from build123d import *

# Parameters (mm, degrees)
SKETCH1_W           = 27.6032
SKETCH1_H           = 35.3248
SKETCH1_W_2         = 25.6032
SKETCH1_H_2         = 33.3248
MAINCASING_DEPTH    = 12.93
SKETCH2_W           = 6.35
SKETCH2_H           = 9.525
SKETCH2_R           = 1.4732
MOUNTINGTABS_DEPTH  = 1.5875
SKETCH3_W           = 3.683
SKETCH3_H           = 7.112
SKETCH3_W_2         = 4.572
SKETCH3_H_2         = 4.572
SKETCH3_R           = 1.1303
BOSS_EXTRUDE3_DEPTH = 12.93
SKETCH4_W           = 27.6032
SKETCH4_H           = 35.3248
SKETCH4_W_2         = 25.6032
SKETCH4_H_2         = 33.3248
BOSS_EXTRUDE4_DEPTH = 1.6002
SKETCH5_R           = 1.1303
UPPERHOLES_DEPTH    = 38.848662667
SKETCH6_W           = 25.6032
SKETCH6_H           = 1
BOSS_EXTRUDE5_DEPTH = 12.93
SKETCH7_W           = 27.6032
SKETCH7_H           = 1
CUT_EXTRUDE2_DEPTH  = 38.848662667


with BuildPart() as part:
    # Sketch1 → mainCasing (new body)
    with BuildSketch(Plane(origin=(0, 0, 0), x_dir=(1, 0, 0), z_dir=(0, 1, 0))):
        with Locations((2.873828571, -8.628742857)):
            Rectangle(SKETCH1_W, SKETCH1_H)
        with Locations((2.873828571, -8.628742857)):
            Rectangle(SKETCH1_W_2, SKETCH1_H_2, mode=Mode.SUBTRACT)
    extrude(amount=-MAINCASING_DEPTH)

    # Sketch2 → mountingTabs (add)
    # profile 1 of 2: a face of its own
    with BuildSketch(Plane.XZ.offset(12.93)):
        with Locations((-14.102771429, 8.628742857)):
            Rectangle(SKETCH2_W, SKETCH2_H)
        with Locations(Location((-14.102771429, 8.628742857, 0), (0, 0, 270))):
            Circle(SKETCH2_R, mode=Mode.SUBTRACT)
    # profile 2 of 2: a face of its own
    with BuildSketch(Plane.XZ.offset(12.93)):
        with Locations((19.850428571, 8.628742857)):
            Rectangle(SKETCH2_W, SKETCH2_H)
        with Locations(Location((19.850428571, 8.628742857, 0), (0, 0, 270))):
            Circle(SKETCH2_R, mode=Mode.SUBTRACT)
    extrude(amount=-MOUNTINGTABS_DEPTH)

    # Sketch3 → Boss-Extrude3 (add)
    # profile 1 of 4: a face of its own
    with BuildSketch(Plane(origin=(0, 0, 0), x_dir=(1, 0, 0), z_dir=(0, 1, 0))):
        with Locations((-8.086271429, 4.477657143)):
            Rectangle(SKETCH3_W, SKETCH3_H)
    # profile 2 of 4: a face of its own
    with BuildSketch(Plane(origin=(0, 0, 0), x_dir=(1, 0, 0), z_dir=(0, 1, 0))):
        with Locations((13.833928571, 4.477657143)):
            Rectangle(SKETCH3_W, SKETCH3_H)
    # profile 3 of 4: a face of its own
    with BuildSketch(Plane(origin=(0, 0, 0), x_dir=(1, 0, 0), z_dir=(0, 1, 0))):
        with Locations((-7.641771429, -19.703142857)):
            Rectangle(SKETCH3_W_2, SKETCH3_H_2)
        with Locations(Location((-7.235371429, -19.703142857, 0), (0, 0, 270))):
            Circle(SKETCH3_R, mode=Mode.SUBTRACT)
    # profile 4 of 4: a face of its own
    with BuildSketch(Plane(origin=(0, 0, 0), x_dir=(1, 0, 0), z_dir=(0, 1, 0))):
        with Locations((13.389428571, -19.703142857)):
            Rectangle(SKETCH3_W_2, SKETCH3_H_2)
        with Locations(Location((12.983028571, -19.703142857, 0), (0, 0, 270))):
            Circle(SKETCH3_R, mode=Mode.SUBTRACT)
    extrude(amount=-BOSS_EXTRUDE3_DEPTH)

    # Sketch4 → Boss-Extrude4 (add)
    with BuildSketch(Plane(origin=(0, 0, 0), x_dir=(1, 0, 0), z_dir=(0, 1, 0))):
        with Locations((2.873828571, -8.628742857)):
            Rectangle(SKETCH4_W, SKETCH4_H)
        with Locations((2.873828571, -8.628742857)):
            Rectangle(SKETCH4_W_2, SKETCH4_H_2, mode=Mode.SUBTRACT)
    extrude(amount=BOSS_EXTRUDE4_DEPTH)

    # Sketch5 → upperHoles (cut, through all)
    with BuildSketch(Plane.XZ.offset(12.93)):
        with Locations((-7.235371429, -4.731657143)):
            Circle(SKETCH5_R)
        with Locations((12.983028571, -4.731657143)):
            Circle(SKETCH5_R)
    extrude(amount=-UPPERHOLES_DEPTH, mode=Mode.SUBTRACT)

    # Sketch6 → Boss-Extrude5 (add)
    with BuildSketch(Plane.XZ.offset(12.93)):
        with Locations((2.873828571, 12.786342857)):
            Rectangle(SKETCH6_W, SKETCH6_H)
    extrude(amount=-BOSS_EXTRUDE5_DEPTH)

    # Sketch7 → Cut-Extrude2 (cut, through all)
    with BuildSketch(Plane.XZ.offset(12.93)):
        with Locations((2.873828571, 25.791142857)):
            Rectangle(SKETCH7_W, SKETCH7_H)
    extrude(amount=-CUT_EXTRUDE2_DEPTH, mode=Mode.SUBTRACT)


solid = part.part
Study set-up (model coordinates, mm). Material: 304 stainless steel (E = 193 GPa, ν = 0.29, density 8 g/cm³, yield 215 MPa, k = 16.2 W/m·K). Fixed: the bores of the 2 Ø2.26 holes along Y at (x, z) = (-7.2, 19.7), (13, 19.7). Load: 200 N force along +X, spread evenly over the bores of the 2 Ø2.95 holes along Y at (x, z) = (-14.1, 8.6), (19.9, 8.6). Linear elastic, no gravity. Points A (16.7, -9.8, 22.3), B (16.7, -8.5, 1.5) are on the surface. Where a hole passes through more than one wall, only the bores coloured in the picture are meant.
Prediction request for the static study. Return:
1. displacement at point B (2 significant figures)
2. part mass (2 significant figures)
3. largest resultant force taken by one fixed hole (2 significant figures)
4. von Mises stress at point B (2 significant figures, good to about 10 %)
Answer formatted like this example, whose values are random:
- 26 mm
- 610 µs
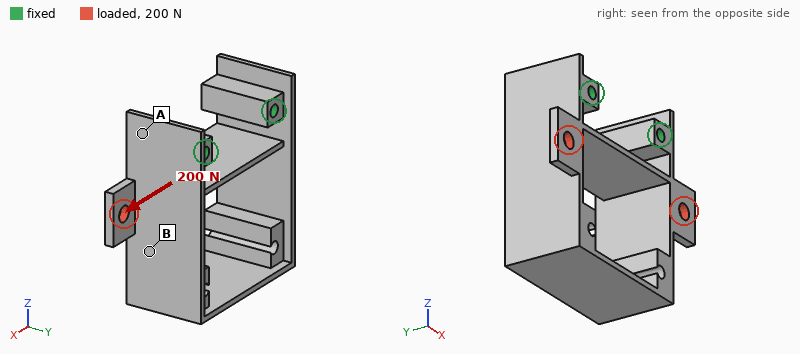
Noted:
- 82 µm
- 23 g
- 120 N
- 69 MPa
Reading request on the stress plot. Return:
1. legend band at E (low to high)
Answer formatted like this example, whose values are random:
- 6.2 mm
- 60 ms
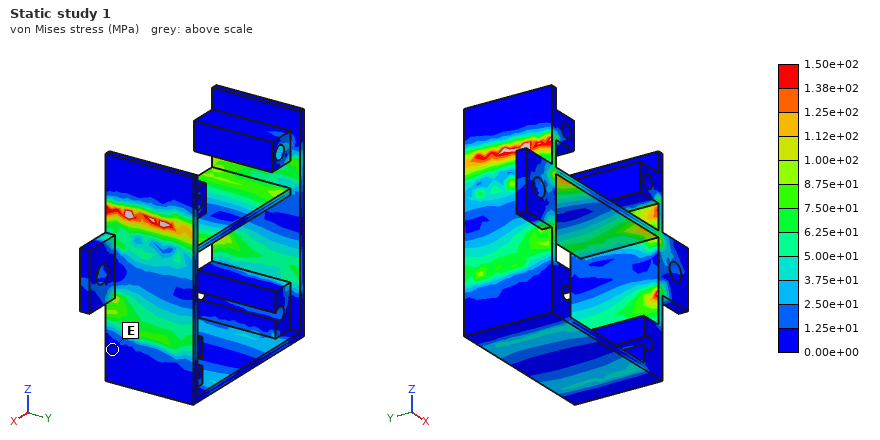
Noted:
- 0.00e+00 to 1.25e+01 MPa
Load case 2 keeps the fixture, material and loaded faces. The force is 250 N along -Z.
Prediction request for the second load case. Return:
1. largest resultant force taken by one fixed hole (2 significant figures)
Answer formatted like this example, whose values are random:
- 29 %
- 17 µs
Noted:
- 140 N
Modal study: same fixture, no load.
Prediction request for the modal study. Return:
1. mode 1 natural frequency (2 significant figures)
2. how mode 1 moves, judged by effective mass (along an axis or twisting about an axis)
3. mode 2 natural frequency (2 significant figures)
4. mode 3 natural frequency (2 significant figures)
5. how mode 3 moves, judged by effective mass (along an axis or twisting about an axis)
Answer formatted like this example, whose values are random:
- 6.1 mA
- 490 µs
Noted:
- 1300 Hz
- along X
- 5000 Hz
- 5400 Hz
- along Y
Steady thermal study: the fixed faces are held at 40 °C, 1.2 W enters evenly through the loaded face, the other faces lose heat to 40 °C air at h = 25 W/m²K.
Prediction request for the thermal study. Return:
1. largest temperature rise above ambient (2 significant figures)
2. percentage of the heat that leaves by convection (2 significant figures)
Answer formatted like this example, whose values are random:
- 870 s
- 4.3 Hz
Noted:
- 27 K
- 56 %
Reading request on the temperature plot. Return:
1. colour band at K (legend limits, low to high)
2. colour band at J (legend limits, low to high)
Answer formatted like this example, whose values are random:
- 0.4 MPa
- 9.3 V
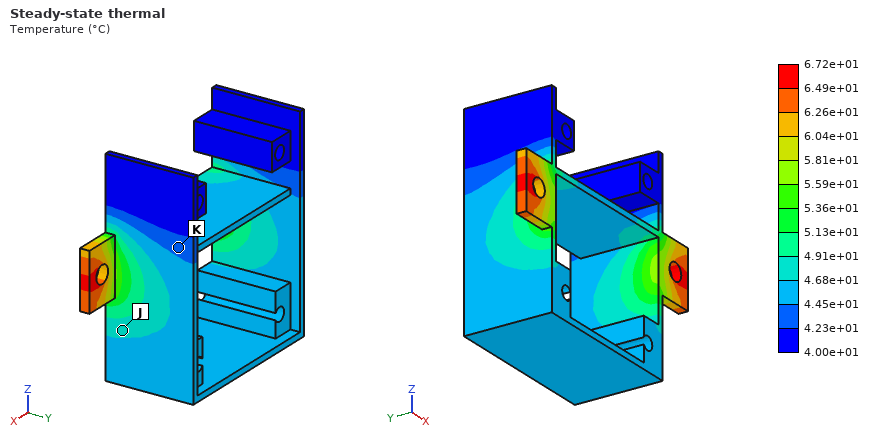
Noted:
- 4.23e+01 to 4.45e+01 °C
- 4.68e+01 to 4.91e+01 °C
